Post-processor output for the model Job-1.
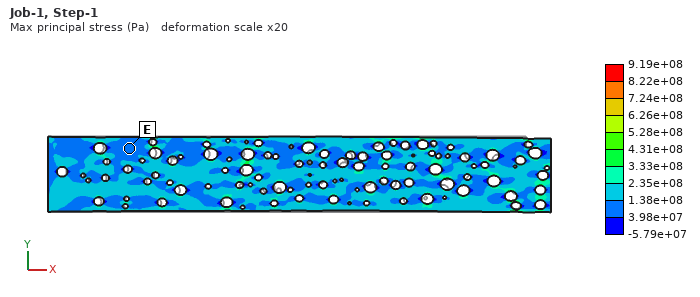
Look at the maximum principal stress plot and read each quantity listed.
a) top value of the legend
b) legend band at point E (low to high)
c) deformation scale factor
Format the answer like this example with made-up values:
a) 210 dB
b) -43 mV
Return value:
a) 9.19e+08 Pa
b) 3.98e+07 to 1.38e+08 Pa
c) 20
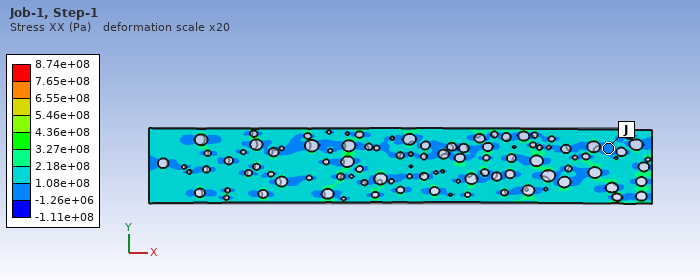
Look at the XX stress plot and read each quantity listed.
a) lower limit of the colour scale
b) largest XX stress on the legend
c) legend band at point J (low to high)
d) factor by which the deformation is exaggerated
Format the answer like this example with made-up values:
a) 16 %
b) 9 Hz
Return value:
a) -1.11e+08 Pa
b) 8.74e+08 Pa
c) -1.26e+06 to 1.08e+08 Pa
d) 20
